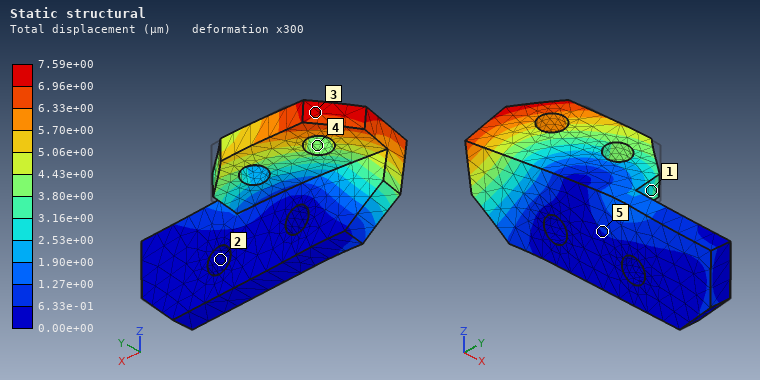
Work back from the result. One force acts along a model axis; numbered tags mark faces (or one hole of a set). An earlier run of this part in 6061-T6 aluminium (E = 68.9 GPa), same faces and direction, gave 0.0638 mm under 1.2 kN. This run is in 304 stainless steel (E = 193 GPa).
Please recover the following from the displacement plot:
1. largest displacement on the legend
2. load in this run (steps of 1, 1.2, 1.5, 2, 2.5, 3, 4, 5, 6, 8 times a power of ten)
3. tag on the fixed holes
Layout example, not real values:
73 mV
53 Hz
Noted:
7.59e+00 µm
400 N
2
